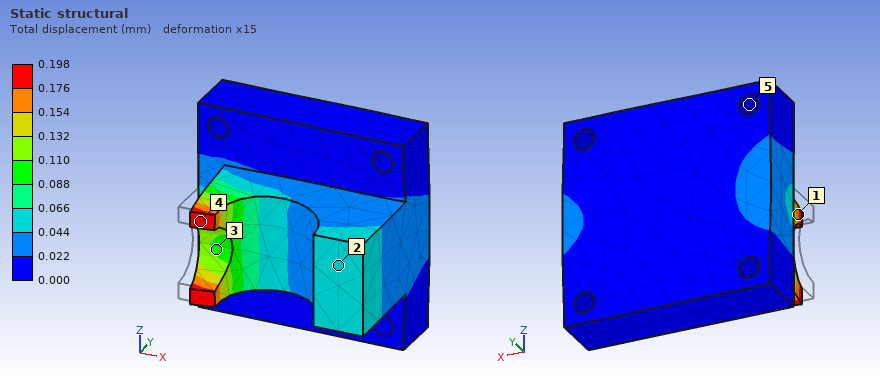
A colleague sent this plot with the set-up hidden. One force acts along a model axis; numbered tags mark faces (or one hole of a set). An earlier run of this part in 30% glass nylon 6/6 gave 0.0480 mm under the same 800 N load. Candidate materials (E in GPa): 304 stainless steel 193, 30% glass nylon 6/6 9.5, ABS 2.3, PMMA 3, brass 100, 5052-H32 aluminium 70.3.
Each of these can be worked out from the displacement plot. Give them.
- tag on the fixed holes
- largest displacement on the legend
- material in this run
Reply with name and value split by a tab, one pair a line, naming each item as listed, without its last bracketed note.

tag on the fixed holes	5
largest displacement on the legend	0.198 mm
material in this run	ABS
